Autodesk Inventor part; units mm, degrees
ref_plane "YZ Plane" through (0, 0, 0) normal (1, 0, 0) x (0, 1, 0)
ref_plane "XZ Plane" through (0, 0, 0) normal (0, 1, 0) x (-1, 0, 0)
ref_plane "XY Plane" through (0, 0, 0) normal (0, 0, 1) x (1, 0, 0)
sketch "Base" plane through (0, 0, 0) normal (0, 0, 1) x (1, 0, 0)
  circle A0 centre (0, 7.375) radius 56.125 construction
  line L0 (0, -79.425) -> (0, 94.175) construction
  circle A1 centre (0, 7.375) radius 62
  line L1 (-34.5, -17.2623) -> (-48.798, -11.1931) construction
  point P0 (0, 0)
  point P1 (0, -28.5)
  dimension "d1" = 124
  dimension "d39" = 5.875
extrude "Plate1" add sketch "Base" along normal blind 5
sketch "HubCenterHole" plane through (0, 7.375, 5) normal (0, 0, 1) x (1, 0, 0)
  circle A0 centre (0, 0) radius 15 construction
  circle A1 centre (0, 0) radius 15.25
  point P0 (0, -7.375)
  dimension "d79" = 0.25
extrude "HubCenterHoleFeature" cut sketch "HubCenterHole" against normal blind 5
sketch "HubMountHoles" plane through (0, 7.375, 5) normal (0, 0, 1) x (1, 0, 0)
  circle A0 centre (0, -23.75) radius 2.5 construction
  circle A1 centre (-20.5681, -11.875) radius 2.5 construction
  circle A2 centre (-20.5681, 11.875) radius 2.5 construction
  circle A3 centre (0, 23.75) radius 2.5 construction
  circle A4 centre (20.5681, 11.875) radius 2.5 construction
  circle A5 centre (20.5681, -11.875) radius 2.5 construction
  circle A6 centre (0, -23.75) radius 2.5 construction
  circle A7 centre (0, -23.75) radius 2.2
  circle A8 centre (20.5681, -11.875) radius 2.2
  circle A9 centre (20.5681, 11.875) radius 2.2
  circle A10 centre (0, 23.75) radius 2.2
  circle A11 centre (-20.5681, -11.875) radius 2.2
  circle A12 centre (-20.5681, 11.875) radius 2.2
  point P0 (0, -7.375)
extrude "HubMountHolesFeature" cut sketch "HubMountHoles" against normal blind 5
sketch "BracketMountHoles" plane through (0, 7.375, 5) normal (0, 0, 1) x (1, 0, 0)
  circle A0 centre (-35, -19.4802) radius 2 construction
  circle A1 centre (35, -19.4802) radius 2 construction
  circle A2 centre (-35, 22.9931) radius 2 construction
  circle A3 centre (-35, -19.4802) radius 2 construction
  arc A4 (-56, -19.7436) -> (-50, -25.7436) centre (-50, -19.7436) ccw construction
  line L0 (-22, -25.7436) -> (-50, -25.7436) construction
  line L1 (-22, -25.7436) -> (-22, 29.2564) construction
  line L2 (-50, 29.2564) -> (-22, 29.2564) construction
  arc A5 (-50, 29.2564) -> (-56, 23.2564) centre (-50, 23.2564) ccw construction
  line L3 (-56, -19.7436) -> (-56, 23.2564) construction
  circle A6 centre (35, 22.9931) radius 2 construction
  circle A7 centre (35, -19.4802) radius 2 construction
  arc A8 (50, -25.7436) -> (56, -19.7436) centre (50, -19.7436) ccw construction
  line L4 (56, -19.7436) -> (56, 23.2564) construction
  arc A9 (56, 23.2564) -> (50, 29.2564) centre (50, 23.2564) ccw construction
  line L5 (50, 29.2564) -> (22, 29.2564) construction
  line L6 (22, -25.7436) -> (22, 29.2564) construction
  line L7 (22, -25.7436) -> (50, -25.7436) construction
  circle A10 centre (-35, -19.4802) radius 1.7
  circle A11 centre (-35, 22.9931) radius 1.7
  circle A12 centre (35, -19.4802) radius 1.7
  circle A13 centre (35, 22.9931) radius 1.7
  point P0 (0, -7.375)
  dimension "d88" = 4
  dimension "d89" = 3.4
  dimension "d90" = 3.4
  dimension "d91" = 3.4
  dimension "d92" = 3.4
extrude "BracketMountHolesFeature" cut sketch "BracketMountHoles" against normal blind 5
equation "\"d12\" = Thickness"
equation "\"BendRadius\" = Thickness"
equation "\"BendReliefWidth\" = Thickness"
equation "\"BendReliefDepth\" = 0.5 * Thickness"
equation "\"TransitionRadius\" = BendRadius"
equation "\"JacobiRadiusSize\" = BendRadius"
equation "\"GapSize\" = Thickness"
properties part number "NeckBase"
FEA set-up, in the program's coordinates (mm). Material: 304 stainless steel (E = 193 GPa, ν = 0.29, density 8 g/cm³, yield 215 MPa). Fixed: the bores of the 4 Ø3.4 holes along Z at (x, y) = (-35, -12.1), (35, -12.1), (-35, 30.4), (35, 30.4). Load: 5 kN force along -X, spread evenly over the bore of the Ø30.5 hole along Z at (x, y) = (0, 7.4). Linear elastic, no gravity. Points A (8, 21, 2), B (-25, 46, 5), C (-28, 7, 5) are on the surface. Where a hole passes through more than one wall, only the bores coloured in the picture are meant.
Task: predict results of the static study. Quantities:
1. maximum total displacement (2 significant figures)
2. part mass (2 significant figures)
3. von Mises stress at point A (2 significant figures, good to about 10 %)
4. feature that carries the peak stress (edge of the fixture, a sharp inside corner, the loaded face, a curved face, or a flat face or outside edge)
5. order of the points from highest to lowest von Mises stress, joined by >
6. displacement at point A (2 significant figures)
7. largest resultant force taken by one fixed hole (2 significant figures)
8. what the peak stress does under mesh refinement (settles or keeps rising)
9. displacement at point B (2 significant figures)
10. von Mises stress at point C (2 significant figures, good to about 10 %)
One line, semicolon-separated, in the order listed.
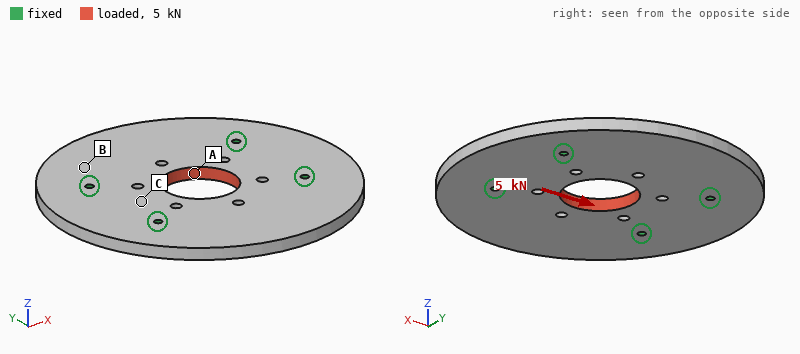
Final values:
2.0 µm; 450 g; 17 MPa; edge of the fixture; A > C > B; 2.0 µm; 1.3 kN; keeps rising; 0.68 µm; 6.6 MPa
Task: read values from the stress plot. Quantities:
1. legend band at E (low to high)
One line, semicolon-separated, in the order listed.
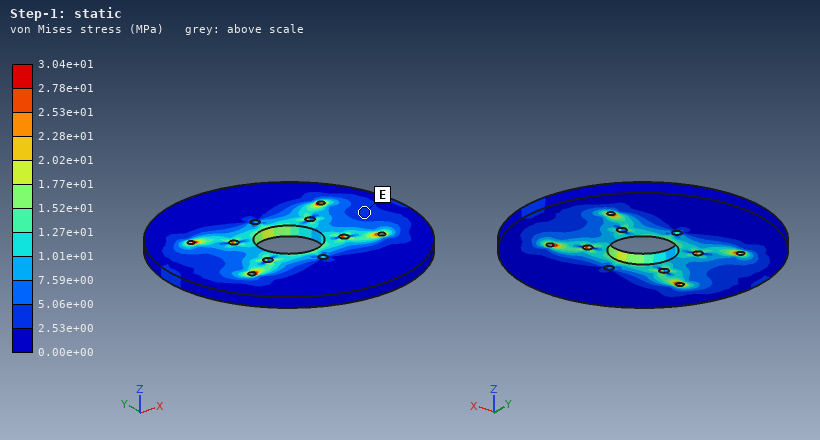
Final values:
2.53e+00 to 5.06e+00 MPa
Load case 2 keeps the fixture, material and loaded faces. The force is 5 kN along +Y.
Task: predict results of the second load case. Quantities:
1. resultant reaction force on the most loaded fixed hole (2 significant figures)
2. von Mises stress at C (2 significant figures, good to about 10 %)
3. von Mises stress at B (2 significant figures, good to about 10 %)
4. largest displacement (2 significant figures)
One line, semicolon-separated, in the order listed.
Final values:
1.3 kN; 8.9 MPa; 6.7 MPa; 3.2 µm
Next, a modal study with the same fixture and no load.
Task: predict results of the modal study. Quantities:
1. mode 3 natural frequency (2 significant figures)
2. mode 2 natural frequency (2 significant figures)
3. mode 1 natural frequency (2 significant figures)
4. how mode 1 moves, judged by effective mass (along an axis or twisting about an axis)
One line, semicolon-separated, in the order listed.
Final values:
4500 Hz; 2300 Hz; 2000 Hz; along Z
